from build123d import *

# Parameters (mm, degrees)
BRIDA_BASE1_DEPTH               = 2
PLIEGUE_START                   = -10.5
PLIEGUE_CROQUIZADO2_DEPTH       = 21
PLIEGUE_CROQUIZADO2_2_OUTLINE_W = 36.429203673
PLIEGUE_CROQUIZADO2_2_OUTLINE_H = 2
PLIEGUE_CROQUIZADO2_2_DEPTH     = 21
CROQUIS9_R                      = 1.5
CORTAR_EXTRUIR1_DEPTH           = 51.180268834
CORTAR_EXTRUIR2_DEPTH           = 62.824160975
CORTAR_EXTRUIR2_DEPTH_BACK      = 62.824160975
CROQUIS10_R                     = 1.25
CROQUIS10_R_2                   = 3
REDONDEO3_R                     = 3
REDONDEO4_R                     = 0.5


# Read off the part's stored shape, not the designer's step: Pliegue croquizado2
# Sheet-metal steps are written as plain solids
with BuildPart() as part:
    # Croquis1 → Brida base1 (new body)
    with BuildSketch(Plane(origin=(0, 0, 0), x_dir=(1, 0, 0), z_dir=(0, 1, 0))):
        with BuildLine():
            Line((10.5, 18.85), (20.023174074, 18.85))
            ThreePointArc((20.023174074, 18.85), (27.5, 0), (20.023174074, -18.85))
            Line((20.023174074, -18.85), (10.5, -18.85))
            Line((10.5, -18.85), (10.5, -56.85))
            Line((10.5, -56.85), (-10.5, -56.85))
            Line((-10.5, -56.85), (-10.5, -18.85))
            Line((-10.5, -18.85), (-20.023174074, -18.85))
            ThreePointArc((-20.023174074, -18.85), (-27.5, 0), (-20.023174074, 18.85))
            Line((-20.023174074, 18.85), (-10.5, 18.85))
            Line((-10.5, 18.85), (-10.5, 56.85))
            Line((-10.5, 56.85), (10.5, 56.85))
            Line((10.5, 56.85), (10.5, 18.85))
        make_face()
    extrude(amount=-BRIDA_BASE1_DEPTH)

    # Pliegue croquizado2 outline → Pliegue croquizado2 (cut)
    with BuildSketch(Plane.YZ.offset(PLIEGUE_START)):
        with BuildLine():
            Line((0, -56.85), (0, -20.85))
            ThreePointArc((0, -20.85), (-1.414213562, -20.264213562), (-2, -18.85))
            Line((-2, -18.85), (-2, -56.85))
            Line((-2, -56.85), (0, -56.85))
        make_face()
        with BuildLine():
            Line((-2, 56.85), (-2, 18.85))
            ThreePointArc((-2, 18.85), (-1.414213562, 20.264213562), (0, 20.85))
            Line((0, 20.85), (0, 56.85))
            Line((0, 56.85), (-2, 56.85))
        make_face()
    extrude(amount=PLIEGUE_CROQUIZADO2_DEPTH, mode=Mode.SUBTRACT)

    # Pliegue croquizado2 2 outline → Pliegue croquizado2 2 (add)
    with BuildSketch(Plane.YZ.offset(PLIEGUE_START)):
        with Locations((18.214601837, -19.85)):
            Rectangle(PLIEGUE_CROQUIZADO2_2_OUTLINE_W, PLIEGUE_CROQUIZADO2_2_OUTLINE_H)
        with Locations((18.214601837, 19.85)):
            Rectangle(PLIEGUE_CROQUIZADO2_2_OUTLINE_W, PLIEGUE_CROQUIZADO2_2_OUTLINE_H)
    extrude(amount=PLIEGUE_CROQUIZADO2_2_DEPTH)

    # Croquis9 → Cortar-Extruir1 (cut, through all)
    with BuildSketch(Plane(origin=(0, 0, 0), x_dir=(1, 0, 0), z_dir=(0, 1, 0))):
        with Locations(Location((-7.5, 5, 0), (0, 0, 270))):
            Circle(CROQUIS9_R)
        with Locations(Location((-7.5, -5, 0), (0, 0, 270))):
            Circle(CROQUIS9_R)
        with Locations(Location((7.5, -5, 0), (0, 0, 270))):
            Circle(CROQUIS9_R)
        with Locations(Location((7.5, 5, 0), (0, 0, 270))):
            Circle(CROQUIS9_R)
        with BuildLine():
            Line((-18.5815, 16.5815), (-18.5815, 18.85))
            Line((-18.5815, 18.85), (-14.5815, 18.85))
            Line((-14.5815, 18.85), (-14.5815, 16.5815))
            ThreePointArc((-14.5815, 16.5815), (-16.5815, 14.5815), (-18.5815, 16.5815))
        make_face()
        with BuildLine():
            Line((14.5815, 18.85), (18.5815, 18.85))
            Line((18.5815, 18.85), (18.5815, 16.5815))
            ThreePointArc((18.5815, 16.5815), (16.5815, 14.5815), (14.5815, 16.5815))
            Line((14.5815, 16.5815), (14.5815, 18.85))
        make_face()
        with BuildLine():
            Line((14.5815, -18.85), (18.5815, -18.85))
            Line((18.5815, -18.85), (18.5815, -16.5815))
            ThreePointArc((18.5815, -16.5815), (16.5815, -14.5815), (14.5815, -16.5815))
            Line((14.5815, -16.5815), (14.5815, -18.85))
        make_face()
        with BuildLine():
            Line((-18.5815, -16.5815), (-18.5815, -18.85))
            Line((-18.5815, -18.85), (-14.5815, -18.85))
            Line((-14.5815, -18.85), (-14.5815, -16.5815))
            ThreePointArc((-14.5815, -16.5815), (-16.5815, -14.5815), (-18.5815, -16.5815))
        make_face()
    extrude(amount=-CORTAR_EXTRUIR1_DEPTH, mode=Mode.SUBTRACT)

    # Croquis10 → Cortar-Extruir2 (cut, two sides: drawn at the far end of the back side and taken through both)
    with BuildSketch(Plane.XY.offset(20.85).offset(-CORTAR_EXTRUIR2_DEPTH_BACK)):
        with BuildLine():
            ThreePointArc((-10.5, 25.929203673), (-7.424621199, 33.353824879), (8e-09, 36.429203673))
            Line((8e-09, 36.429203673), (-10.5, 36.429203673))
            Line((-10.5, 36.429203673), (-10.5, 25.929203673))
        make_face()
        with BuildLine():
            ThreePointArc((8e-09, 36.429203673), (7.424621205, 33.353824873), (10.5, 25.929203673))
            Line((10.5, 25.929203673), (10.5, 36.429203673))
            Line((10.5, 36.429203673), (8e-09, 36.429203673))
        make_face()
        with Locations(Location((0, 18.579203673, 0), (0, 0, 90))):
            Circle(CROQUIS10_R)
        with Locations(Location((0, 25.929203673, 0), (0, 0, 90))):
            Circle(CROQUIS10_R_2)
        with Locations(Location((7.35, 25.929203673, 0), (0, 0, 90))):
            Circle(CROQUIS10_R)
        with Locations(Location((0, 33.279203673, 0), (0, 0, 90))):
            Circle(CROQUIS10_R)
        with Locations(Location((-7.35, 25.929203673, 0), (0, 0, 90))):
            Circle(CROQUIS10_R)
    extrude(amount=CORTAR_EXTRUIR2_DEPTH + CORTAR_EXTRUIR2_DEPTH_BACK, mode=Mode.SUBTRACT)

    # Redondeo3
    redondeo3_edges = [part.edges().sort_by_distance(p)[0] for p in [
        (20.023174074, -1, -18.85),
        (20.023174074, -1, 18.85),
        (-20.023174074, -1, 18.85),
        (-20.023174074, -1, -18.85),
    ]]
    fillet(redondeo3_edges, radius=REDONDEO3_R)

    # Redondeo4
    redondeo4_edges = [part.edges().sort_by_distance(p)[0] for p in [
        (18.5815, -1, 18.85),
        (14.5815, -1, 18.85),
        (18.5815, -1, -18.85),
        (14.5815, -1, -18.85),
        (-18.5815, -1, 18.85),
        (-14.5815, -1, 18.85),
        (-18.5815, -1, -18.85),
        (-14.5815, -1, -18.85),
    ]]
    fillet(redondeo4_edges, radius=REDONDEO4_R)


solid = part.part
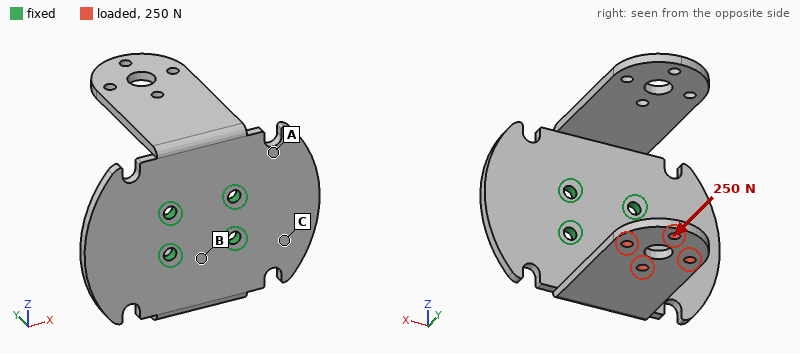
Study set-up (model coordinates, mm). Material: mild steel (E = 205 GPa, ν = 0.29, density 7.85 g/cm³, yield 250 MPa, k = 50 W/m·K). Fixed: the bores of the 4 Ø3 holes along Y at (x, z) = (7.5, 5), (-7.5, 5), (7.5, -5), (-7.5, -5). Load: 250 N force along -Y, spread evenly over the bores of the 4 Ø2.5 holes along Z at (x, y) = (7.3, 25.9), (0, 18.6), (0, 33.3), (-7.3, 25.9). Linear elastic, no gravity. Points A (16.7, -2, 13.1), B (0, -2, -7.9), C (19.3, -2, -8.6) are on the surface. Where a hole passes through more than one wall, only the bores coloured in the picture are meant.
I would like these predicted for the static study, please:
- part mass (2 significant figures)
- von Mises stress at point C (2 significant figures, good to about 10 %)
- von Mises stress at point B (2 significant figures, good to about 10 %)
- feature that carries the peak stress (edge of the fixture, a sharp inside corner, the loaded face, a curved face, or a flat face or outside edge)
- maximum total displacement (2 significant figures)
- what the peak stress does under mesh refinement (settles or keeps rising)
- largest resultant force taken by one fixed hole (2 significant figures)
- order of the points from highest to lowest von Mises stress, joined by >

50 g
41 MPa
93 MPa
edge of the fixture
0.22 mm
keeps rising
180 N
B > C > A
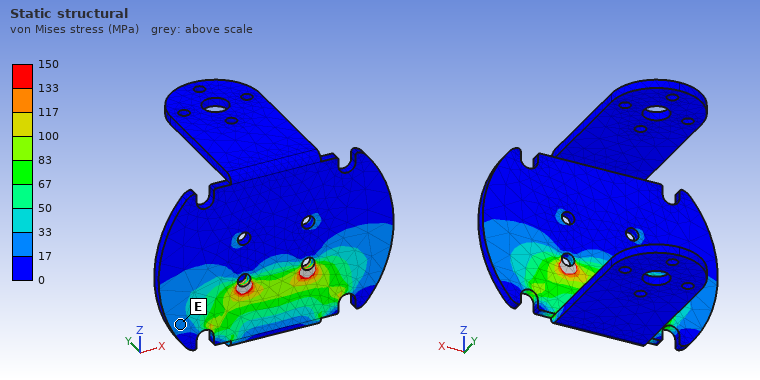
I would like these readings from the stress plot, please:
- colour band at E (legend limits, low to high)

17 to 33 MPa
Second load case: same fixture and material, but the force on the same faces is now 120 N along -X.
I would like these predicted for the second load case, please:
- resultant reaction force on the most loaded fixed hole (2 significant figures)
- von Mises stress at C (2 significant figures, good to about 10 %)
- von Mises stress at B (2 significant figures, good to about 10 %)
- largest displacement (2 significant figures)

230 N
33 MPa
36 MPa
0.14 mm
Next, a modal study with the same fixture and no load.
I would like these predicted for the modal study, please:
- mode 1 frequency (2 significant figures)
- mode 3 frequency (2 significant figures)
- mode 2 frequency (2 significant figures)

970 Hz
2100 Hz
970 Hz
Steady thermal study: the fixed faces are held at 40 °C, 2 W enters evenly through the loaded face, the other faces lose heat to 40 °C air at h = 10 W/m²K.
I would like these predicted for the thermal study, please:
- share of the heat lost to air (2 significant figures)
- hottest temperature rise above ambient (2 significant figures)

21 %
34 K
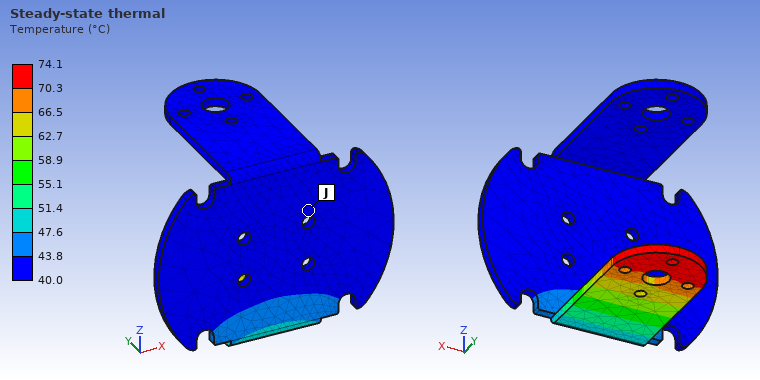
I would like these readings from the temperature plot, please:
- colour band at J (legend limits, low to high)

40.0 to 43.8 °C
